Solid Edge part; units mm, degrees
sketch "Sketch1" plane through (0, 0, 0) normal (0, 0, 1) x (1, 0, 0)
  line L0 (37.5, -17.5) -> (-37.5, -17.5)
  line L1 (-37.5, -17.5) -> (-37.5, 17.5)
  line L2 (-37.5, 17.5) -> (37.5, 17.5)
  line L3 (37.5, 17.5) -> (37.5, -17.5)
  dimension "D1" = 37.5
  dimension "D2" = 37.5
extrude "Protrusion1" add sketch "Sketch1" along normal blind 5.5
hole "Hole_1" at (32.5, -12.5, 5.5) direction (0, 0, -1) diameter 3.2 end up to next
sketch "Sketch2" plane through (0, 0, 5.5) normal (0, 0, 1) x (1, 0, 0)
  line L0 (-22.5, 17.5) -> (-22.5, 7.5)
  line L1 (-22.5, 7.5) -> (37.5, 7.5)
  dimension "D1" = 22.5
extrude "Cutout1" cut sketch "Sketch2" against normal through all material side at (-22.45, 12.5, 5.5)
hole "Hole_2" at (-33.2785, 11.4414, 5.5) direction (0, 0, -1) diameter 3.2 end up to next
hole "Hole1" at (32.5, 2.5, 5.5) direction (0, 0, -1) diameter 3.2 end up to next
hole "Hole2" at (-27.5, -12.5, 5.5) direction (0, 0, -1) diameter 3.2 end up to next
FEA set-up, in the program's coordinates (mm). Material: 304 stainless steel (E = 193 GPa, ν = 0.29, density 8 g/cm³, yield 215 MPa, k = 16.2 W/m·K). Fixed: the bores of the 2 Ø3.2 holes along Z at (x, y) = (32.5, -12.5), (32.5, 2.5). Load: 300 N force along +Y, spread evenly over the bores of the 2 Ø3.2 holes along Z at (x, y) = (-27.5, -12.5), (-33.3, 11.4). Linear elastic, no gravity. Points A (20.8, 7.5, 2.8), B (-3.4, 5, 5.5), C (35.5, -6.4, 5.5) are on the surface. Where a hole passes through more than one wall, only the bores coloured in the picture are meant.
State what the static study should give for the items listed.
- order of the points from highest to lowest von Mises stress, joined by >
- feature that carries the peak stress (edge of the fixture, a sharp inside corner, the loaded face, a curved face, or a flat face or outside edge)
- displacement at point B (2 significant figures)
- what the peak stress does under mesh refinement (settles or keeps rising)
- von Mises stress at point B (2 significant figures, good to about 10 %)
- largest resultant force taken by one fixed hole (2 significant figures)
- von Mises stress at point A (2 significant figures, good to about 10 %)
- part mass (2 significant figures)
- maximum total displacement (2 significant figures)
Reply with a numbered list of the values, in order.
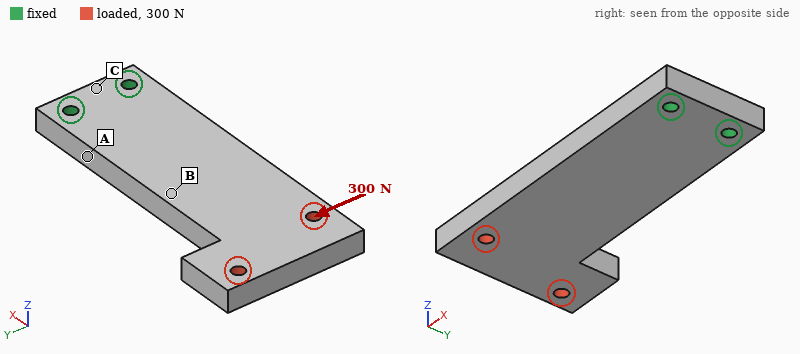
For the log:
1. A > B > C
2. edge of the fixture
3. 9.7 µm
4. keeps rising
5. 11 MPa
6. 1.1 kN
7. 26 MPa
8. 88 g
9. 27 µm
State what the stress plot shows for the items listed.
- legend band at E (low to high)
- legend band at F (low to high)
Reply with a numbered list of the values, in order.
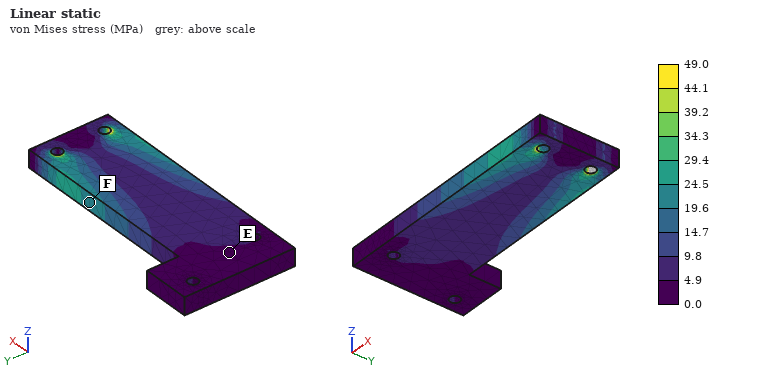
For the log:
1. 0.0 to 4.9 MPa
2. 19.6 to 24.5 MPa
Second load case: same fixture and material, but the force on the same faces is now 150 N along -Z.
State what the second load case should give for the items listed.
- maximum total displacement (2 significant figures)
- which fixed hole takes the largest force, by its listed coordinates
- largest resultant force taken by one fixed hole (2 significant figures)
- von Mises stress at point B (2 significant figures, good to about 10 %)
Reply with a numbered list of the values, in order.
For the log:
1. 0.23 mm
2. (32.5, 2.5)
3. 110 N
4. 32 MPa
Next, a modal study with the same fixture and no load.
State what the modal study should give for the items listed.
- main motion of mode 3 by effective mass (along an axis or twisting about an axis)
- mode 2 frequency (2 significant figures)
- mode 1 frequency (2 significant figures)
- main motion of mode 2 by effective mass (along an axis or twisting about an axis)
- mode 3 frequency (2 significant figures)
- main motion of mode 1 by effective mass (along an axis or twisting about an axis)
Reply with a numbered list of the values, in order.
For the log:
1. twisting about X
2. 3200 Hz
3. 800 Hz
4. along Y
5. 3500 Hz
6. along Z
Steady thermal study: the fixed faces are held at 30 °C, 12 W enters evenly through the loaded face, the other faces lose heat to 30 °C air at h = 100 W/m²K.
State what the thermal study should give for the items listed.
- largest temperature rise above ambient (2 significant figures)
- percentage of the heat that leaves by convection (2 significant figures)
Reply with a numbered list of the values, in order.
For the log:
1. 78 K
2. 96 %
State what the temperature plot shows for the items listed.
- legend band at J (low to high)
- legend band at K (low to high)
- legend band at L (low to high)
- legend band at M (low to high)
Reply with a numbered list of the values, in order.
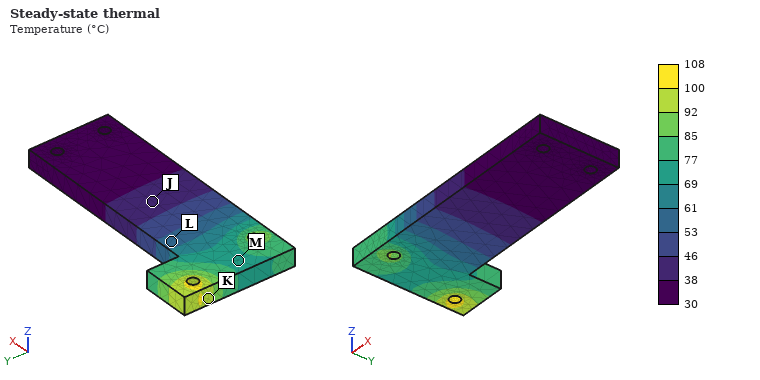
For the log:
1. 38 to 46 °C
2. 92 to 100 °C
3. 53 to 61 °C
4. 69 to 77 °C
